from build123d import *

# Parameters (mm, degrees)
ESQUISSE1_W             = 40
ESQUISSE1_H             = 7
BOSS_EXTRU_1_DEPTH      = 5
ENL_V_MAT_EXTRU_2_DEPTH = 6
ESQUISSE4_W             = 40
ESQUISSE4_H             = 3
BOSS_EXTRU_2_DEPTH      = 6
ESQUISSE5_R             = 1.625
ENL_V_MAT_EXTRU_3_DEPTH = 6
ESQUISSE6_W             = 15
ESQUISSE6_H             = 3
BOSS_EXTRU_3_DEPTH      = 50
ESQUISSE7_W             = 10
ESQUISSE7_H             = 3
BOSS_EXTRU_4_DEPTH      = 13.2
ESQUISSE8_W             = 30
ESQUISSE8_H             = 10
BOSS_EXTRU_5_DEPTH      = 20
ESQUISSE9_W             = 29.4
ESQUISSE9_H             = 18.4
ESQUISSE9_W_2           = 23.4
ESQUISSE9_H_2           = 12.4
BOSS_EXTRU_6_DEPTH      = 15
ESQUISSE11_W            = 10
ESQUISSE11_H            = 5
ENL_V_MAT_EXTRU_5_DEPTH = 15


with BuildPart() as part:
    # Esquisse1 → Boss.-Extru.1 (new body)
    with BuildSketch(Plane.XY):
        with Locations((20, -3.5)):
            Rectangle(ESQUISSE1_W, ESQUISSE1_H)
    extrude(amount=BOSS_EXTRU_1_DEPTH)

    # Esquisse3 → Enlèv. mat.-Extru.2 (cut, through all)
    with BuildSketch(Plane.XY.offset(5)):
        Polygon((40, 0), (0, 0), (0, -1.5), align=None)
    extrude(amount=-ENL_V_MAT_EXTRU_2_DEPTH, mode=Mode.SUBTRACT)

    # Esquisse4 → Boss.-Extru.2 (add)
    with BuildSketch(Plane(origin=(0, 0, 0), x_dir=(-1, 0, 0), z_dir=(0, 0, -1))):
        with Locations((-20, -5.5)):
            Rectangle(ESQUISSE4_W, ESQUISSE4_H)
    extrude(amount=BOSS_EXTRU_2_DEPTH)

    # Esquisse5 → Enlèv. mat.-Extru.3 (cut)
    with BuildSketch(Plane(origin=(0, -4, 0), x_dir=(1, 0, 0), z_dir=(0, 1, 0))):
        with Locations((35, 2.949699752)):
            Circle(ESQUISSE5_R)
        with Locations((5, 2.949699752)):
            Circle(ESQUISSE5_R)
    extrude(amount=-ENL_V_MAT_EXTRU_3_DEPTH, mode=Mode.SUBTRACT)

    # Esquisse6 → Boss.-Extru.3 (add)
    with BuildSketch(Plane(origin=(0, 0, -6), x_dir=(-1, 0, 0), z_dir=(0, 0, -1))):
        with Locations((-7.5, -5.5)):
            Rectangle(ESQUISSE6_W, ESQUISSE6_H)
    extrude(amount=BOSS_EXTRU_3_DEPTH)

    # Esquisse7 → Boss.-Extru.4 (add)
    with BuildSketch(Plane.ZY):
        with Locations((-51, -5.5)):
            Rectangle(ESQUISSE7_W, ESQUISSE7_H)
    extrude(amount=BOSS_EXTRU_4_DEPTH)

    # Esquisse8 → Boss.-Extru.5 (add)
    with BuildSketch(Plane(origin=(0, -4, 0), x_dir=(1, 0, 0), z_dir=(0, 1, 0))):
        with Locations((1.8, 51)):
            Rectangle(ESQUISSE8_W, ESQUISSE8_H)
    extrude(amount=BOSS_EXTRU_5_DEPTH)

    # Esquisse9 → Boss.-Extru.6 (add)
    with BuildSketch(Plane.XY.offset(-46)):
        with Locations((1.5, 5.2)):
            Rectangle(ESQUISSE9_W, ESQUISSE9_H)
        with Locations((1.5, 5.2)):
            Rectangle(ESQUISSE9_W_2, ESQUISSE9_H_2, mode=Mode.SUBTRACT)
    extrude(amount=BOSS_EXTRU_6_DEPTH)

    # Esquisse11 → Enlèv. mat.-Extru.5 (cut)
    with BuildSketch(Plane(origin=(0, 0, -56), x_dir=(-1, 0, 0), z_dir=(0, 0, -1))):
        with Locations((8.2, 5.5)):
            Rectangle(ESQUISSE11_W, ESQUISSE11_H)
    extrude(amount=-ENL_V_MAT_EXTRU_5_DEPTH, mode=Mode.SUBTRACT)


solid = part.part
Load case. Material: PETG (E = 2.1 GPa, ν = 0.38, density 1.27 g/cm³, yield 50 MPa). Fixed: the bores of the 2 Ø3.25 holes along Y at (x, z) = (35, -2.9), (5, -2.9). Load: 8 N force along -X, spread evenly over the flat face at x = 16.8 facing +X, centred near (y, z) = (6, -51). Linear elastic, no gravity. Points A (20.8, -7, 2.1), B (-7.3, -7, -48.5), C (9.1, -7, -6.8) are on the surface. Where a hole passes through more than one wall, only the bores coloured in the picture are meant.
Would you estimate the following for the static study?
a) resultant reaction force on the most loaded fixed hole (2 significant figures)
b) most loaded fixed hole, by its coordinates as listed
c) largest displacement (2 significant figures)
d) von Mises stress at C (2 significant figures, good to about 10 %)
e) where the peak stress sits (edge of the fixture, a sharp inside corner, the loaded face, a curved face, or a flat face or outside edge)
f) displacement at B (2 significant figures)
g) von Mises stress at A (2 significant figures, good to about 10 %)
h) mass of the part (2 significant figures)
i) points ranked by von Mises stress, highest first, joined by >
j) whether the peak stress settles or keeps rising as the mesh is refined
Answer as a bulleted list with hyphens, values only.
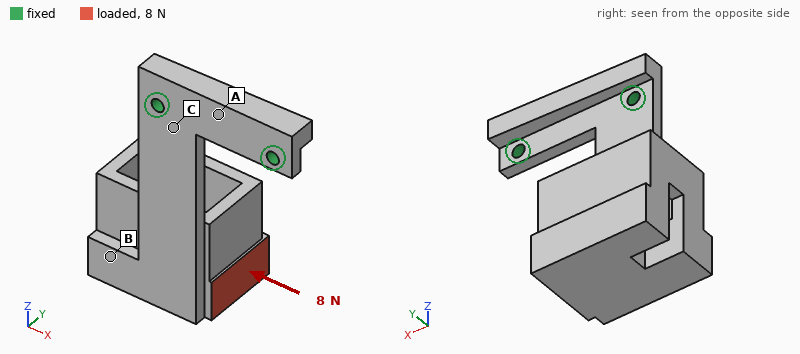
- 18 N
- (5, -2.9)
- 0.94 mm
- 2.7 MPa
- edge of the fixture
- 0.39 mm
- 1.3 MPa
- 17 g
- C > A > B
- keeps rising
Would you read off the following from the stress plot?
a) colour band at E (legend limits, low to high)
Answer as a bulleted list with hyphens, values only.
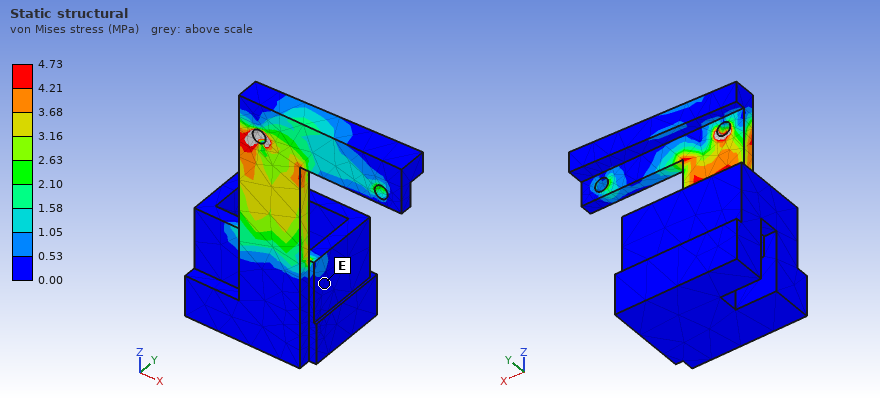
- 0.00 to 0.53 MPa
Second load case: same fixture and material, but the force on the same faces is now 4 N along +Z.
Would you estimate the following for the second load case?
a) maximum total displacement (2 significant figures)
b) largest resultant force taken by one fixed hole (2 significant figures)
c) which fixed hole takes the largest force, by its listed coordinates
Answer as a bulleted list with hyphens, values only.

- 0.82 mm
- 2.8 N
- (5, -2.9)
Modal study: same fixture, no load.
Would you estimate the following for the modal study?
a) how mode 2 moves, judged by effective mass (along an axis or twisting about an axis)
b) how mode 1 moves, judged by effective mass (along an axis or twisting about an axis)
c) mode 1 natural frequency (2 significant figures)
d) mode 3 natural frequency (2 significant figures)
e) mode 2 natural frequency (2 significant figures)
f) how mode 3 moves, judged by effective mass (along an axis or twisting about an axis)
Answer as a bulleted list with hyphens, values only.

- along X
- along Y
- 67 Hz
- 370 Hz
- 160 Hz
- along X
